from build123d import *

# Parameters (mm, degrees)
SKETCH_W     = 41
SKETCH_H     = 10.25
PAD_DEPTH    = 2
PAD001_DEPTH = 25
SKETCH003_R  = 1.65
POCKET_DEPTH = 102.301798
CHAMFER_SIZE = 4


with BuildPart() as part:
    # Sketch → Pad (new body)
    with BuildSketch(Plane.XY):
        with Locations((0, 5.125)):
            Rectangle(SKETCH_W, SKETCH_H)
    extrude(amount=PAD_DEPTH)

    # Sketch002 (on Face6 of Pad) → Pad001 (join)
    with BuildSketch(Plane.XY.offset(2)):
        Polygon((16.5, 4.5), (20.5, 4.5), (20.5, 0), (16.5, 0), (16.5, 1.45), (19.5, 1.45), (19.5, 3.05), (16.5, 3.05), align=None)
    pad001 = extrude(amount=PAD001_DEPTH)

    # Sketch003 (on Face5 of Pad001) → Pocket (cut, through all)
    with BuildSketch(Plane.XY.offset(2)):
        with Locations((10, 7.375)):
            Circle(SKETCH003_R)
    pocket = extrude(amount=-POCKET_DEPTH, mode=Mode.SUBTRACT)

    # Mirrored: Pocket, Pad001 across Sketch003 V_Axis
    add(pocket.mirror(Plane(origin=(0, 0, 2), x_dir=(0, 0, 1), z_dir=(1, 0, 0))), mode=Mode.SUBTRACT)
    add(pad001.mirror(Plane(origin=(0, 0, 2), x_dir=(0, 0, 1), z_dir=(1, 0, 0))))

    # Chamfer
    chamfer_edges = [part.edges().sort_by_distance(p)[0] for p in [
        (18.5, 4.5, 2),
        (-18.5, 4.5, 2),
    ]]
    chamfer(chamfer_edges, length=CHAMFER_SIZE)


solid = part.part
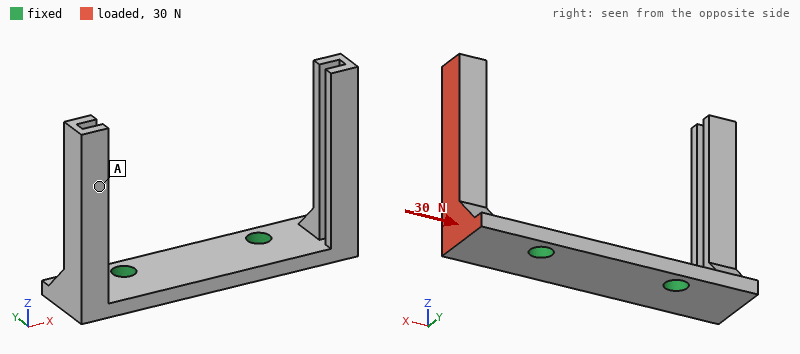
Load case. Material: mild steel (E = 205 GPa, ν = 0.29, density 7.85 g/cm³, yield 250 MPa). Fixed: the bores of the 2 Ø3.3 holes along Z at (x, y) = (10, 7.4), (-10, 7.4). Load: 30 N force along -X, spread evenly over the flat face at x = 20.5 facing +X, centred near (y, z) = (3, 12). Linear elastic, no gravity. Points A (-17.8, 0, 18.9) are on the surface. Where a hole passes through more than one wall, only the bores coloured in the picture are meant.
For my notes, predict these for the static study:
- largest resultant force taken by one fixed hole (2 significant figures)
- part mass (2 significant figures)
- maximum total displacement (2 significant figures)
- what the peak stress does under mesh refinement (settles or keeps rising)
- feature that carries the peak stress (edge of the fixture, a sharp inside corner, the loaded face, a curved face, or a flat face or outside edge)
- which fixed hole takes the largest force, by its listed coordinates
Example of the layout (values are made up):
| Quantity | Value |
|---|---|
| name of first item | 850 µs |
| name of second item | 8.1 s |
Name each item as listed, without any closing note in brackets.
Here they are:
| Quantity | Value |
|---|---|
| largest resultant force taken by one fixed hole | 23 N |
| part mass | 12 g |
| maximum total displacement | 57 µm |
| what the peak stress does under mesh refinement | keeps rising |
| feature that carries the peak stress | edge of the fixture |
| which fixed hole takes the largest force, by its listed coordinates | (10, 7.4) |
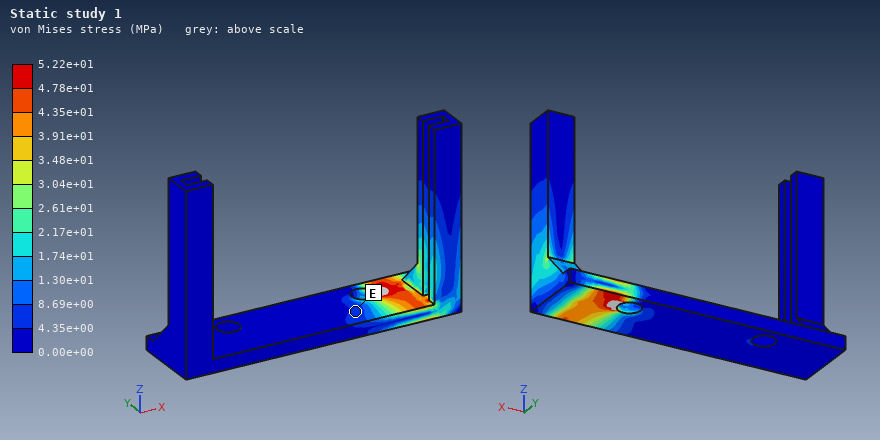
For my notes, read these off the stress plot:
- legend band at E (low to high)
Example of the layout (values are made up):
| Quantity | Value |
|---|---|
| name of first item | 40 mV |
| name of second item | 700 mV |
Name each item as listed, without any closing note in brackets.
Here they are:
| Quantity | Value |
|---|---|
| legend band at E | 4.35e+00 to 8.69e+00 MPa |
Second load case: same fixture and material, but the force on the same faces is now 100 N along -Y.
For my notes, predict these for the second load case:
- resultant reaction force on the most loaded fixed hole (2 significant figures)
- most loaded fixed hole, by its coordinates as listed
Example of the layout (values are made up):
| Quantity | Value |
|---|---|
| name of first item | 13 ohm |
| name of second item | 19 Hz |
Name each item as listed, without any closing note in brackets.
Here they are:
| Quantity | Value |
|---|---|
| resultant reaction force on the most loaded fixed hole | 130 N |
| most loaded fixed hole, by its coordinates as listed | (10, 7.4) |
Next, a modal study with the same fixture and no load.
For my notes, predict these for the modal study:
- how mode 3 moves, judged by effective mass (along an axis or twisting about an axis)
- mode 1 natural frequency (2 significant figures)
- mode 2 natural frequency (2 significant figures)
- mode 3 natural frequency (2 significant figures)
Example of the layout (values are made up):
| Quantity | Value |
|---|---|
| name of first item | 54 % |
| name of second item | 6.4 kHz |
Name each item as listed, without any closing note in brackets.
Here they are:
| Quantity | Value |
|---|---|
| how mode 3 moves, judged by effective mass | along Y |
| mode 1 natural frequency | 2400 Hz |
| mode 2 natural frequency | 2400 Hz |
| mode 3 natural frequency | 3200 Hz |
